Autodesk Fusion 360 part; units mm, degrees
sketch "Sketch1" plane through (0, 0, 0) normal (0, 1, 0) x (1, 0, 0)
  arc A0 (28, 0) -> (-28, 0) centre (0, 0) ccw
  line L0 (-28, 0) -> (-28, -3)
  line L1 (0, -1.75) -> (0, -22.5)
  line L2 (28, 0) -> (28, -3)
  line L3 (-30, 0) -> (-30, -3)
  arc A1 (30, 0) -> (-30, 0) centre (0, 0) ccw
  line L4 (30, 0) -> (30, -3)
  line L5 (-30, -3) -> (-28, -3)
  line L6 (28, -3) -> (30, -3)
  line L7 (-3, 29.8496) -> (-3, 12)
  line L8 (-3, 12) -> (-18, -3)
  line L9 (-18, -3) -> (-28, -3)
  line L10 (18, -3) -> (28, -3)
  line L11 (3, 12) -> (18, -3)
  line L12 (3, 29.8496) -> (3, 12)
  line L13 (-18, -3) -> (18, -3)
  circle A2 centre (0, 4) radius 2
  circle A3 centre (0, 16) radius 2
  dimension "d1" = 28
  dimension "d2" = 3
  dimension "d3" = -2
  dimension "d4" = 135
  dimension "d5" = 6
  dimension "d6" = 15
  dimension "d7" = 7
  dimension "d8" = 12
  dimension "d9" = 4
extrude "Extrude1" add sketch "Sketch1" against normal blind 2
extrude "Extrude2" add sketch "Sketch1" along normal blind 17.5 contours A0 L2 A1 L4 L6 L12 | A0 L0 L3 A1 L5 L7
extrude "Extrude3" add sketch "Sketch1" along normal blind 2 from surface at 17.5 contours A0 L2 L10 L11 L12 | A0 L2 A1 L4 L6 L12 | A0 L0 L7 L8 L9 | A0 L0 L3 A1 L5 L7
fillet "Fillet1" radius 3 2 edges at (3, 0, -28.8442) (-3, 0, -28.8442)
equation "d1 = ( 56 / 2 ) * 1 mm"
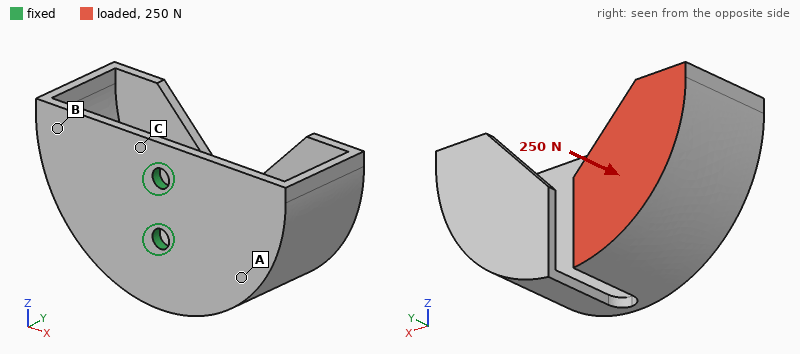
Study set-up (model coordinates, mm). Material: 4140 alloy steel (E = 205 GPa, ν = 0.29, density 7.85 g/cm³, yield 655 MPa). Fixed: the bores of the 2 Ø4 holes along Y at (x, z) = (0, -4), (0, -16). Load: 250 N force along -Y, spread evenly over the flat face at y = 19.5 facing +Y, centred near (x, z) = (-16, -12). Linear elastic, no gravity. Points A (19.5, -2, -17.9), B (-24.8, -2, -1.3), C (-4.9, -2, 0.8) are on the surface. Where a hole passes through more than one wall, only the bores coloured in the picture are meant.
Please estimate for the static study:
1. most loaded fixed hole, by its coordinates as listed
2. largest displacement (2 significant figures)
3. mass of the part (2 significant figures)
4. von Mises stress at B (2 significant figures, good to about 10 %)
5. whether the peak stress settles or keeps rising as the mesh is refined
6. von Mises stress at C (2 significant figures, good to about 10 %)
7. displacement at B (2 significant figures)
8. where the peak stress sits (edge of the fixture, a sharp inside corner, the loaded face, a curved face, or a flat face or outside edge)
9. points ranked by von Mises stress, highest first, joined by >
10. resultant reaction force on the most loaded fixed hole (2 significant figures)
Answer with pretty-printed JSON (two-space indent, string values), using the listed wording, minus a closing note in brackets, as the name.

{
  "most loaded fixed hole, by its coordinates as listed": "(0, -16)",
  "largest displacement": "0.18 mm",
  "mass of the part": "68 g",
  "von Mises stress at B": "46 MPa",
  "whether the peak stress settles or keeps rising as the mesh is refined": "keeps rising",
  "von Mises stress at C": "110 MPa",
  "displacement at B": "0.12 mm",
  "where the peak stress sits": "edge of the fixture",
  "points ranked by von Mises stress, highest first, joined by >": "C > B > A",
  "resultant reaction force on the most loaded fixed hole": "160 N"
}
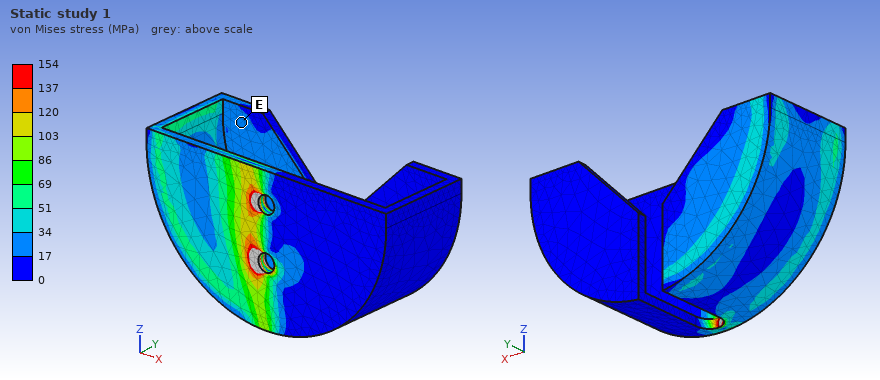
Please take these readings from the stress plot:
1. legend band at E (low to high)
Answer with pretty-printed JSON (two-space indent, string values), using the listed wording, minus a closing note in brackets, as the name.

{
  "legend band at E": "17 to 34 MPa"
}
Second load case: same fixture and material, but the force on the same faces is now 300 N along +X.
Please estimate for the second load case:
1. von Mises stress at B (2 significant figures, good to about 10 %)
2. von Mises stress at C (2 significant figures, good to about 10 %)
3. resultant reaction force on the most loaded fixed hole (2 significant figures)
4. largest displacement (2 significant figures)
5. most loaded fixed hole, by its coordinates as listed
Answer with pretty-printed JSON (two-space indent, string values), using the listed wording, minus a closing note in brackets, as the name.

{
  "von Mises stress at B": "120 MPa",
  "von Mises stress at C": "140 MPa",
  "resultant reaction force on the most loaded fixed hole": "200 N",
  "largest displacement": "0.50 mm",
  "most loaded fixed hole, by its coordinates as listed": "(0, -16)"
}
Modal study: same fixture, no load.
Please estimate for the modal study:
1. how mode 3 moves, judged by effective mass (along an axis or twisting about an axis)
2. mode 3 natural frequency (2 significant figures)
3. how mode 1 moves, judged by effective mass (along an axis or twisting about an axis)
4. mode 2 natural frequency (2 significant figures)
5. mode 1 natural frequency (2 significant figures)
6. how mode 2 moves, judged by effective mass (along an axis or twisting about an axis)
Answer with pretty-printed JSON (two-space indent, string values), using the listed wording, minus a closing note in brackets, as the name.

{
  "how mode 3 moves, judged by effective mass": "along Z",
  "mode 3 natural frequency": "1300 Hz",
  "how mode 1 moves, judged by effective mass": "along X",
  "mode 2 natural frequency": "1100 Hz",
  "mode 1 natural frequency": "920 Hz",
  "how mode 2 moves, judged by effective mass": "along Y"
}
